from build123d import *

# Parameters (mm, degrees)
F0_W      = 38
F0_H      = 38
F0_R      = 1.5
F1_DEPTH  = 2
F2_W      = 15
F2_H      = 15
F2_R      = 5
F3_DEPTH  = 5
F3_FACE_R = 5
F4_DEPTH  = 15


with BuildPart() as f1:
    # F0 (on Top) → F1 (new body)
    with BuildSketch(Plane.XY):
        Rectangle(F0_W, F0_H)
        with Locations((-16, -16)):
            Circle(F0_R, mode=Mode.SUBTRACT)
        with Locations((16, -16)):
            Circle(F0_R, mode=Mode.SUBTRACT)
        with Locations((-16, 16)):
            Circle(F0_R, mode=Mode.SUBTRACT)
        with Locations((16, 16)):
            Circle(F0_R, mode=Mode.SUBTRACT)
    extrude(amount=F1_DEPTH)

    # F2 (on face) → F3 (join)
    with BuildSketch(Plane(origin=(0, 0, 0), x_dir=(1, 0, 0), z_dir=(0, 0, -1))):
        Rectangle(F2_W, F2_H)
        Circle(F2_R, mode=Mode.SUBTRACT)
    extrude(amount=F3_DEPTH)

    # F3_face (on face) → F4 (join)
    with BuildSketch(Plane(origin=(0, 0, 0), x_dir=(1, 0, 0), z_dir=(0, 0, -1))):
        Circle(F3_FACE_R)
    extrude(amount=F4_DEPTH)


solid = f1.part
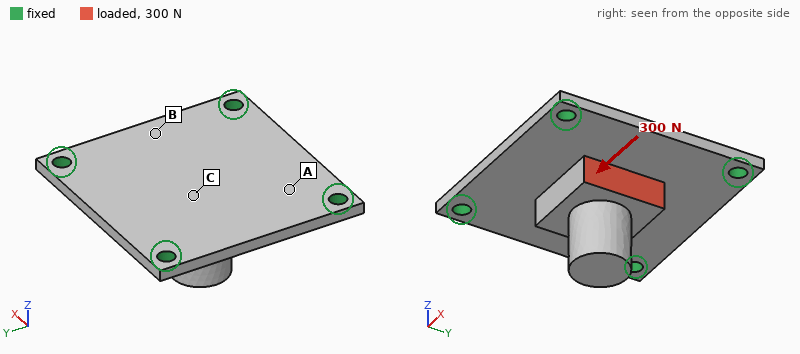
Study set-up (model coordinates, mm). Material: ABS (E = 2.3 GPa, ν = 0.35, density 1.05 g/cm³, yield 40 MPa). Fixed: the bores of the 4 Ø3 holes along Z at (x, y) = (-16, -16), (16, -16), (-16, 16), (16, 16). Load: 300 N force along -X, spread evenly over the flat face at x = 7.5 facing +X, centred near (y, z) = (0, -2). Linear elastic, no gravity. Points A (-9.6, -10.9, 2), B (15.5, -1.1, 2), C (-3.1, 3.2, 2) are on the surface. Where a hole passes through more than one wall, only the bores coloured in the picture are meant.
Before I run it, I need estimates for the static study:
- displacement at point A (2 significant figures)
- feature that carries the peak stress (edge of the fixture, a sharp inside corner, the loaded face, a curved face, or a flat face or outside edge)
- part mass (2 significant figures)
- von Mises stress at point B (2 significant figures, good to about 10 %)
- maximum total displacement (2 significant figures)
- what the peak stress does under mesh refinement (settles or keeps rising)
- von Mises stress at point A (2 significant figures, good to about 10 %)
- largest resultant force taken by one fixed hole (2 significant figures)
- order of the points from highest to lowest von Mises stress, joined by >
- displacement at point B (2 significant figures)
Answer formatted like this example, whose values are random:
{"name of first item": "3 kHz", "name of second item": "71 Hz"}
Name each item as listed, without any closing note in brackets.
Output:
{"displacement at point A": "0.084 mm", "feature that carries the peak stress": "edge of the fixture", "part mass": "5.0 g", "von Mises stress at point B": "6.5 MPa", "maximum total displacement": "0.34 mm", "what the peak stress does under mesh refinement": "keeps rising", "von Mises stress at point A": "4.0 MPa", "largest resultant force taken by one fixed hole": "88 N", "order of the points from highest to lowest von Mises stress, joined by >": "B > A > C", "displacement at point B": "0.17 mm"}
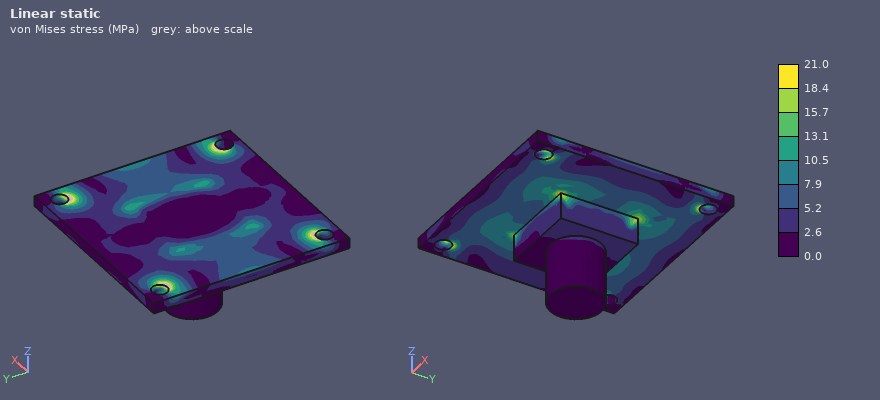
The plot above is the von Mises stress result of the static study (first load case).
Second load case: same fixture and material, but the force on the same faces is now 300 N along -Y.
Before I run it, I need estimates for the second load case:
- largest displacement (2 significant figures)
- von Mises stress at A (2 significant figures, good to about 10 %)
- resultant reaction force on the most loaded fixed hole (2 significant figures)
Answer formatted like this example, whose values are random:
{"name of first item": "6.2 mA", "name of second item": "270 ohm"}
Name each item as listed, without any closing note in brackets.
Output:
{"largest displacement": "0.34 mm", "von Mises stress at A": "3.9 MPa", "resultant reaction force on the most loaded fixed hole": "100 N"}
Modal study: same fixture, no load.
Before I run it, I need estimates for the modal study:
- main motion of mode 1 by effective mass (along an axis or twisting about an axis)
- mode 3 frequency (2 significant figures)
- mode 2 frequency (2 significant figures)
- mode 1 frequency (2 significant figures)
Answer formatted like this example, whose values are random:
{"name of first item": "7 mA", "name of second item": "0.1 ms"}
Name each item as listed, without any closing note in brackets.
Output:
{"main motion of mode 1 by effective mass": "along Z", "mode 3 frequency": "2400 Hz", "mode 2 frequency": "2400 Hz", "mode 1 frequency": "1700 Hz"}
